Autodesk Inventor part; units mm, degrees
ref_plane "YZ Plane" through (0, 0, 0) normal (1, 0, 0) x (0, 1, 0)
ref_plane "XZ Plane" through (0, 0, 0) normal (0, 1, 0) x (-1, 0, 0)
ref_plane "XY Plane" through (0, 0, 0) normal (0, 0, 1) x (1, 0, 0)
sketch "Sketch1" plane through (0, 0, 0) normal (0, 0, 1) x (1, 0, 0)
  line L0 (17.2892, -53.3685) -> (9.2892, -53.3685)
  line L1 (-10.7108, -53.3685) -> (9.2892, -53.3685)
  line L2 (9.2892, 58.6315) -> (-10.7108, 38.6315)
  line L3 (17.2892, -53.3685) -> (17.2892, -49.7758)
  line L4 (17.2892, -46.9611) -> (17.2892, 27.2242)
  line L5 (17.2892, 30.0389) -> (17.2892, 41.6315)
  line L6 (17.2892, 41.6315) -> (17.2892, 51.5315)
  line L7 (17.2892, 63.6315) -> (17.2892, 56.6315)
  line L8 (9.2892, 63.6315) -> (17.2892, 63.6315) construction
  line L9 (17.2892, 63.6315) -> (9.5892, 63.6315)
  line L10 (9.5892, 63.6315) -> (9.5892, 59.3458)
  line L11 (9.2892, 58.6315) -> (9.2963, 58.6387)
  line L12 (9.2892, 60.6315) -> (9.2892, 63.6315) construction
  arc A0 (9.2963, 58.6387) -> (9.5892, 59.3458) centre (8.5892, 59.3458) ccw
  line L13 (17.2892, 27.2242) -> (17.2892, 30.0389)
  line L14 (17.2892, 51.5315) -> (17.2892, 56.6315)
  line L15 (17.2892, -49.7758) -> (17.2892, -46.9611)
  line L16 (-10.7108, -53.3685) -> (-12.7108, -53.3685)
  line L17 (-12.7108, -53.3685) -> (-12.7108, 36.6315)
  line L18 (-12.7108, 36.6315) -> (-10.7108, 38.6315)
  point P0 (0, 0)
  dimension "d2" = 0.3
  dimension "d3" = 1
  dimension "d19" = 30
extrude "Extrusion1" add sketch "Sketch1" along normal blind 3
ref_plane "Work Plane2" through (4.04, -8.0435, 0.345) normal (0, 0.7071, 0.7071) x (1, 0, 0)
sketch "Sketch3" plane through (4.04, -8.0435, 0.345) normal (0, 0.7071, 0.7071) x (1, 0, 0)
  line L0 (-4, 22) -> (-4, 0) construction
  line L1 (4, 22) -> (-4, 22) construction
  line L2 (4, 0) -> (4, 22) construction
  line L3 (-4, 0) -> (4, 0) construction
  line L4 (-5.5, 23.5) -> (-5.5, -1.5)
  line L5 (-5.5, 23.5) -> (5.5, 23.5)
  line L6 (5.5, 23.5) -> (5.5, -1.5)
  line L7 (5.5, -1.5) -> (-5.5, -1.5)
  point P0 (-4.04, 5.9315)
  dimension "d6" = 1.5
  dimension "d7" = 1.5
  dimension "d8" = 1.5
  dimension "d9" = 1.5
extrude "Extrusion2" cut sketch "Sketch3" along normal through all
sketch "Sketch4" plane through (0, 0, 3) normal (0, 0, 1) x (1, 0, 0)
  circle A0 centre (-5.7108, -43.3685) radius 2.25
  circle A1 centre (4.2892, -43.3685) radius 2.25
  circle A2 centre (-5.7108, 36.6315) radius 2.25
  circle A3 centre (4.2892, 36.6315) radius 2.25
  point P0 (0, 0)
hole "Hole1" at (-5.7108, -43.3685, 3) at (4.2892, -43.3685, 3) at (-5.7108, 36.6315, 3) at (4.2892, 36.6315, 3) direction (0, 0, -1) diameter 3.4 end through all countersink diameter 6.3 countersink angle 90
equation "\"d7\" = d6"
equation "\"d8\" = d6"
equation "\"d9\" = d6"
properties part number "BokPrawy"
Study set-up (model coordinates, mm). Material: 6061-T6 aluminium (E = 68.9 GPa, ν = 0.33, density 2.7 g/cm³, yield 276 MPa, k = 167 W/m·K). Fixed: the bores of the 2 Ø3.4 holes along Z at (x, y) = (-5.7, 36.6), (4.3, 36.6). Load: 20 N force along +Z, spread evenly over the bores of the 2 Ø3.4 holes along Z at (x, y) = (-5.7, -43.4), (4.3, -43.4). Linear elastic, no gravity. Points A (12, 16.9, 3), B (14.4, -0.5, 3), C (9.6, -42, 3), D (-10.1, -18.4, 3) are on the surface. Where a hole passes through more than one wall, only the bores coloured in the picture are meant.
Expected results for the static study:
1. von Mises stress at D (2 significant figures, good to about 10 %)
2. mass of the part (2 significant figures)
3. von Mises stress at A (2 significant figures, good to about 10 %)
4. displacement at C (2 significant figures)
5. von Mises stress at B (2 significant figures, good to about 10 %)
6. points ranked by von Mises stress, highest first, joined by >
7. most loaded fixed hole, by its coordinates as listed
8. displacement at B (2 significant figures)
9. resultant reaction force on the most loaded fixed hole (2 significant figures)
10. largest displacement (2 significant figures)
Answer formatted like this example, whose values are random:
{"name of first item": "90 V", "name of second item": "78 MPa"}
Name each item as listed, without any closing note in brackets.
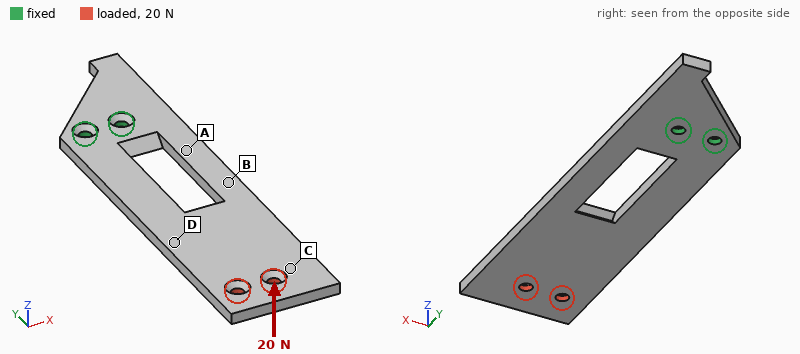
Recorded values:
{"von Mises stress at D": "12 MPa", "mass of the part": "22 g", "von Mises stress at A": "42 MPa", "displacement at C": "1.1 mm", "von Mises stress at B": "31 MPa", "points ranked by von Mises stress, highest first, joined by >": "A > B > D > C", "most loaded fixed hole, by its coordinates as listed": "(-5.7, 36.6)", "displacement at B": "0.31 mm", "resultant reaction force on the most loaded fixed hole": "22 N", "largest displacement": "1.3 mm"}
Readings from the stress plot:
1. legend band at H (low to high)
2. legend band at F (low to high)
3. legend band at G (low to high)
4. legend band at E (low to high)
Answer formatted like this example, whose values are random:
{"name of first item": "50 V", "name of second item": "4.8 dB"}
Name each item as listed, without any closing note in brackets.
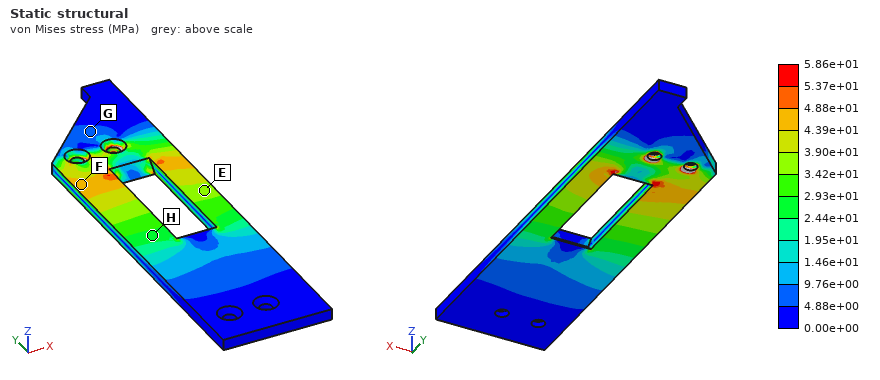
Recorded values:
{"legend band at H": "2.44e+01 to 2.93e+01 MPa", "legend band at F": "4.39e+01 to 4.88e+01 MPa", "legend band at G": "4.88e+00 to 9.76e+00 MPa", "legend band at E": "3.42e+01 to 3.90e+01 MPa"}
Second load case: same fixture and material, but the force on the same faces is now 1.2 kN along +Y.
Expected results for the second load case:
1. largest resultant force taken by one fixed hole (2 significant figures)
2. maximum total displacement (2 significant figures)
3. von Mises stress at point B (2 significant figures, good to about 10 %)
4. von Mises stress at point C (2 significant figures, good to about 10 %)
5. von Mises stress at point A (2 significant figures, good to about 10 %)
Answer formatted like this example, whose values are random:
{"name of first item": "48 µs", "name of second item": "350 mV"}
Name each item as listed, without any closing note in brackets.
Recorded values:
{"largest resultant force taken by one fixed hole": "610 N", "maximum total displacement": "1.0 mm", "von Mises stress at point B": "16 MPa", "von Mises stress at point C": "6.9 MPa", "von Mises stress at point A": "11 MPa"}
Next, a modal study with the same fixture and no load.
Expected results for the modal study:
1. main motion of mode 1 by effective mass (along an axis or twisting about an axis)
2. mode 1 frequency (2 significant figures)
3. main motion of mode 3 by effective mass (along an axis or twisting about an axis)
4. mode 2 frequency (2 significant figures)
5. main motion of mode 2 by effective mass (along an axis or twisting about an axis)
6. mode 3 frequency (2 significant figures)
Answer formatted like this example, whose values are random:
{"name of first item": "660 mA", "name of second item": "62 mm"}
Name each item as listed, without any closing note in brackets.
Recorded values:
{"main motion of mode 1 by effective mass": "along Z", "mode 1 frequency": "250 Hz", "main motion of mode 3 by effective mass": "along X", "mode 2 frequency": "1400 Hz", "main motion of mode 2 by effective mass": "twisting about Y", "mode 3 frequency": "1700 Hz"}
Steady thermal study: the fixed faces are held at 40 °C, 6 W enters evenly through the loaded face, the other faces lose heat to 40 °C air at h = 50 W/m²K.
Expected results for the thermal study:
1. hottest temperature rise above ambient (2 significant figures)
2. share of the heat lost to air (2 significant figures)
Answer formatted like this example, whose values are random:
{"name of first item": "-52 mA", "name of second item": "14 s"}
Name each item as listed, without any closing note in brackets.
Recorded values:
{"hottest temperature rise above ambient": "25 K", "share of the heat lost to air": "59 %"}
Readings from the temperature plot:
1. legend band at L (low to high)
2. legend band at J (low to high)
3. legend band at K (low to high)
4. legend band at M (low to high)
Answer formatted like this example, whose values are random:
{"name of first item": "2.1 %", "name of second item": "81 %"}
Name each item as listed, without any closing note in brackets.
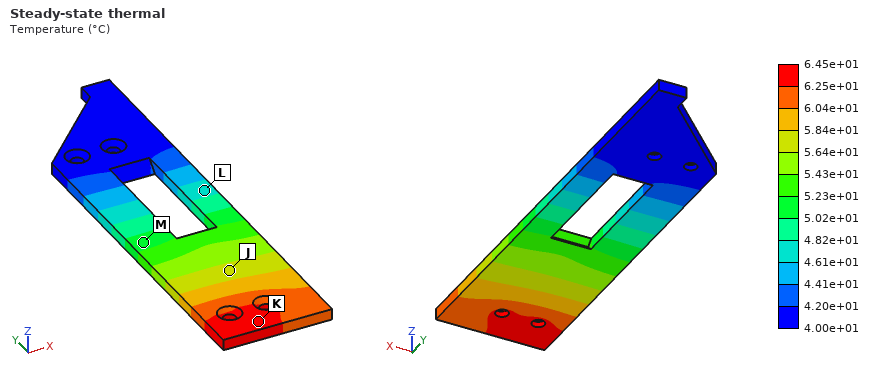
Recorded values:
{"legend band at L": "4.61e+01 to 4.82e+01 °C", "legend band at J": "5.64e+01 to 5.84e+01 °C", "legend band at K": "6.25e+01 to 6.45e+01 °C", "legend band at M": "5.02e+01 to 5.23e+01 °C"}
